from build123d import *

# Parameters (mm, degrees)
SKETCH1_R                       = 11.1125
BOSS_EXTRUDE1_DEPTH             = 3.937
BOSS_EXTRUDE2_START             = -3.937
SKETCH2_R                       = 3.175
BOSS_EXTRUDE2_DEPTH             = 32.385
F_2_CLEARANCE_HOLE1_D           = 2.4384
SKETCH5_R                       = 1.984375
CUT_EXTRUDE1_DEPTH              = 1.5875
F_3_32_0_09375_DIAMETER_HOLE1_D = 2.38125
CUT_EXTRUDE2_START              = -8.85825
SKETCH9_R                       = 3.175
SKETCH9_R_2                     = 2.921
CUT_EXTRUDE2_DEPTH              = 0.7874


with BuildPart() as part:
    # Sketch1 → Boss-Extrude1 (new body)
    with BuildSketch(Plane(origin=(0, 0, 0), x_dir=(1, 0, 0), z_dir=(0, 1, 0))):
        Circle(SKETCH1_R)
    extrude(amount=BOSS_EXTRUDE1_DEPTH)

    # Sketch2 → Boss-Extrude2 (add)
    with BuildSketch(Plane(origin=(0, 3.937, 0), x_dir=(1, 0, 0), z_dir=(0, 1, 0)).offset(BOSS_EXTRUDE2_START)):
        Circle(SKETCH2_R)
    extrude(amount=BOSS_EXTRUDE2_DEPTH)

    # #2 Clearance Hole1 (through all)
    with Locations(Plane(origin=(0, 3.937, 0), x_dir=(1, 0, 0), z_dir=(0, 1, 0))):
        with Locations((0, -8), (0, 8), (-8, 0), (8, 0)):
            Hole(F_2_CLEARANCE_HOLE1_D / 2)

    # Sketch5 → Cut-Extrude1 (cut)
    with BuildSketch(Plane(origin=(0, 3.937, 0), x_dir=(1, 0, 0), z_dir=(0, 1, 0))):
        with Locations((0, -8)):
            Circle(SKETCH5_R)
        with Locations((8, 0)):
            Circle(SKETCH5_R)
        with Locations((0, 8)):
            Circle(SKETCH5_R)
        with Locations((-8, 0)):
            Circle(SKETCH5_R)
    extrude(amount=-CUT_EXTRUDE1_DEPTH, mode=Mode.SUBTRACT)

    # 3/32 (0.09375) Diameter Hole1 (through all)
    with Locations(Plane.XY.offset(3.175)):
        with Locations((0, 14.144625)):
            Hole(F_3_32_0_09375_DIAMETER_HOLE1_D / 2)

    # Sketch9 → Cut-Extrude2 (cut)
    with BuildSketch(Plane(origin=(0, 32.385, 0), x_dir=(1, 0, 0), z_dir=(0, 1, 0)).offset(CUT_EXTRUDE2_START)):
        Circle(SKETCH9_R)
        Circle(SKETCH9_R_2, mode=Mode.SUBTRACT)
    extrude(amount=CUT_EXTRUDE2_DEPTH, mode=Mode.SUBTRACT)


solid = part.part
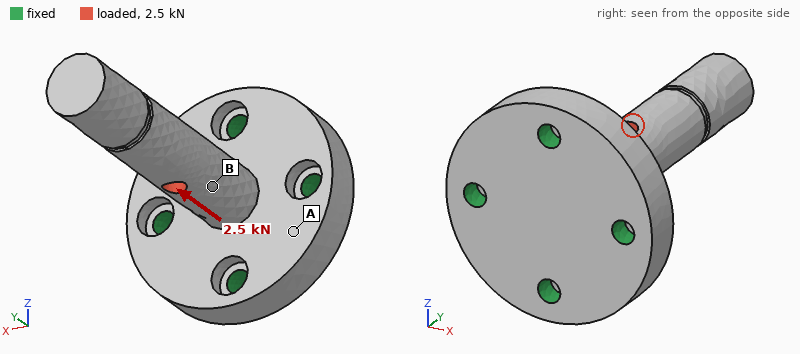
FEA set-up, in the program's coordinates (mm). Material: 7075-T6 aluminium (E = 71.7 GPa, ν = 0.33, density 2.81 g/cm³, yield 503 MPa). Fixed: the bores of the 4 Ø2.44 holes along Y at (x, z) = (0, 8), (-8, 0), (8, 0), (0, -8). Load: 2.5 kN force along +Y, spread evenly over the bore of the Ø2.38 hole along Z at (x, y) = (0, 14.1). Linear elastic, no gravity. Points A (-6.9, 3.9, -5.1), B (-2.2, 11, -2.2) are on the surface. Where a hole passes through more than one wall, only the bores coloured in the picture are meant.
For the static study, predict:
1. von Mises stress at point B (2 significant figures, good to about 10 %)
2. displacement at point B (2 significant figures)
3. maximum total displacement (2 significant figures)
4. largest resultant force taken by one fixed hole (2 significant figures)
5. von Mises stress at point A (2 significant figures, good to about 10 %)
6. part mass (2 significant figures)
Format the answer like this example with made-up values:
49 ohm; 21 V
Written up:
84 MPa; 18 µm; 25 µm; 730 N; 20 MPa; 6.4 g
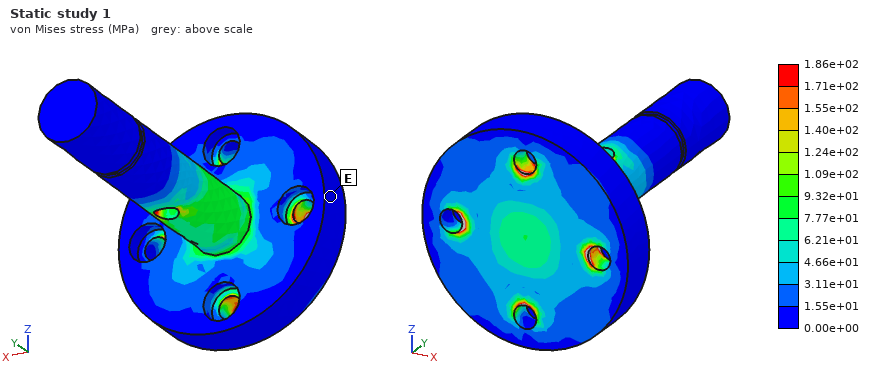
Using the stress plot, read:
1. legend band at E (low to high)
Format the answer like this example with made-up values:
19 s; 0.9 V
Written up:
0.00e+00 to 1.55e+01 MPa
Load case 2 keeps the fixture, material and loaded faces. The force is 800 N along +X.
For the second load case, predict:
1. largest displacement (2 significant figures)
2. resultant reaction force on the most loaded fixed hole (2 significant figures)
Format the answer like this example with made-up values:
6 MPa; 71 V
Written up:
0.28 mm; 780 N
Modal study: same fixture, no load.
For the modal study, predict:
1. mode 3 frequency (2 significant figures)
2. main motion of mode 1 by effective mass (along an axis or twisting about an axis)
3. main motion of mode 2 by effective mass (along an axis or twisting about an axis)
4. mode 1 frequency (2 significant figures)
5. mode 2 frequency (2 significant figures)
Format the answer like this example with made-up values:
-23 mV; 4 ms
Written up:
25 kHz; along Z; along X; 4500 Hz; 4700 Hz
